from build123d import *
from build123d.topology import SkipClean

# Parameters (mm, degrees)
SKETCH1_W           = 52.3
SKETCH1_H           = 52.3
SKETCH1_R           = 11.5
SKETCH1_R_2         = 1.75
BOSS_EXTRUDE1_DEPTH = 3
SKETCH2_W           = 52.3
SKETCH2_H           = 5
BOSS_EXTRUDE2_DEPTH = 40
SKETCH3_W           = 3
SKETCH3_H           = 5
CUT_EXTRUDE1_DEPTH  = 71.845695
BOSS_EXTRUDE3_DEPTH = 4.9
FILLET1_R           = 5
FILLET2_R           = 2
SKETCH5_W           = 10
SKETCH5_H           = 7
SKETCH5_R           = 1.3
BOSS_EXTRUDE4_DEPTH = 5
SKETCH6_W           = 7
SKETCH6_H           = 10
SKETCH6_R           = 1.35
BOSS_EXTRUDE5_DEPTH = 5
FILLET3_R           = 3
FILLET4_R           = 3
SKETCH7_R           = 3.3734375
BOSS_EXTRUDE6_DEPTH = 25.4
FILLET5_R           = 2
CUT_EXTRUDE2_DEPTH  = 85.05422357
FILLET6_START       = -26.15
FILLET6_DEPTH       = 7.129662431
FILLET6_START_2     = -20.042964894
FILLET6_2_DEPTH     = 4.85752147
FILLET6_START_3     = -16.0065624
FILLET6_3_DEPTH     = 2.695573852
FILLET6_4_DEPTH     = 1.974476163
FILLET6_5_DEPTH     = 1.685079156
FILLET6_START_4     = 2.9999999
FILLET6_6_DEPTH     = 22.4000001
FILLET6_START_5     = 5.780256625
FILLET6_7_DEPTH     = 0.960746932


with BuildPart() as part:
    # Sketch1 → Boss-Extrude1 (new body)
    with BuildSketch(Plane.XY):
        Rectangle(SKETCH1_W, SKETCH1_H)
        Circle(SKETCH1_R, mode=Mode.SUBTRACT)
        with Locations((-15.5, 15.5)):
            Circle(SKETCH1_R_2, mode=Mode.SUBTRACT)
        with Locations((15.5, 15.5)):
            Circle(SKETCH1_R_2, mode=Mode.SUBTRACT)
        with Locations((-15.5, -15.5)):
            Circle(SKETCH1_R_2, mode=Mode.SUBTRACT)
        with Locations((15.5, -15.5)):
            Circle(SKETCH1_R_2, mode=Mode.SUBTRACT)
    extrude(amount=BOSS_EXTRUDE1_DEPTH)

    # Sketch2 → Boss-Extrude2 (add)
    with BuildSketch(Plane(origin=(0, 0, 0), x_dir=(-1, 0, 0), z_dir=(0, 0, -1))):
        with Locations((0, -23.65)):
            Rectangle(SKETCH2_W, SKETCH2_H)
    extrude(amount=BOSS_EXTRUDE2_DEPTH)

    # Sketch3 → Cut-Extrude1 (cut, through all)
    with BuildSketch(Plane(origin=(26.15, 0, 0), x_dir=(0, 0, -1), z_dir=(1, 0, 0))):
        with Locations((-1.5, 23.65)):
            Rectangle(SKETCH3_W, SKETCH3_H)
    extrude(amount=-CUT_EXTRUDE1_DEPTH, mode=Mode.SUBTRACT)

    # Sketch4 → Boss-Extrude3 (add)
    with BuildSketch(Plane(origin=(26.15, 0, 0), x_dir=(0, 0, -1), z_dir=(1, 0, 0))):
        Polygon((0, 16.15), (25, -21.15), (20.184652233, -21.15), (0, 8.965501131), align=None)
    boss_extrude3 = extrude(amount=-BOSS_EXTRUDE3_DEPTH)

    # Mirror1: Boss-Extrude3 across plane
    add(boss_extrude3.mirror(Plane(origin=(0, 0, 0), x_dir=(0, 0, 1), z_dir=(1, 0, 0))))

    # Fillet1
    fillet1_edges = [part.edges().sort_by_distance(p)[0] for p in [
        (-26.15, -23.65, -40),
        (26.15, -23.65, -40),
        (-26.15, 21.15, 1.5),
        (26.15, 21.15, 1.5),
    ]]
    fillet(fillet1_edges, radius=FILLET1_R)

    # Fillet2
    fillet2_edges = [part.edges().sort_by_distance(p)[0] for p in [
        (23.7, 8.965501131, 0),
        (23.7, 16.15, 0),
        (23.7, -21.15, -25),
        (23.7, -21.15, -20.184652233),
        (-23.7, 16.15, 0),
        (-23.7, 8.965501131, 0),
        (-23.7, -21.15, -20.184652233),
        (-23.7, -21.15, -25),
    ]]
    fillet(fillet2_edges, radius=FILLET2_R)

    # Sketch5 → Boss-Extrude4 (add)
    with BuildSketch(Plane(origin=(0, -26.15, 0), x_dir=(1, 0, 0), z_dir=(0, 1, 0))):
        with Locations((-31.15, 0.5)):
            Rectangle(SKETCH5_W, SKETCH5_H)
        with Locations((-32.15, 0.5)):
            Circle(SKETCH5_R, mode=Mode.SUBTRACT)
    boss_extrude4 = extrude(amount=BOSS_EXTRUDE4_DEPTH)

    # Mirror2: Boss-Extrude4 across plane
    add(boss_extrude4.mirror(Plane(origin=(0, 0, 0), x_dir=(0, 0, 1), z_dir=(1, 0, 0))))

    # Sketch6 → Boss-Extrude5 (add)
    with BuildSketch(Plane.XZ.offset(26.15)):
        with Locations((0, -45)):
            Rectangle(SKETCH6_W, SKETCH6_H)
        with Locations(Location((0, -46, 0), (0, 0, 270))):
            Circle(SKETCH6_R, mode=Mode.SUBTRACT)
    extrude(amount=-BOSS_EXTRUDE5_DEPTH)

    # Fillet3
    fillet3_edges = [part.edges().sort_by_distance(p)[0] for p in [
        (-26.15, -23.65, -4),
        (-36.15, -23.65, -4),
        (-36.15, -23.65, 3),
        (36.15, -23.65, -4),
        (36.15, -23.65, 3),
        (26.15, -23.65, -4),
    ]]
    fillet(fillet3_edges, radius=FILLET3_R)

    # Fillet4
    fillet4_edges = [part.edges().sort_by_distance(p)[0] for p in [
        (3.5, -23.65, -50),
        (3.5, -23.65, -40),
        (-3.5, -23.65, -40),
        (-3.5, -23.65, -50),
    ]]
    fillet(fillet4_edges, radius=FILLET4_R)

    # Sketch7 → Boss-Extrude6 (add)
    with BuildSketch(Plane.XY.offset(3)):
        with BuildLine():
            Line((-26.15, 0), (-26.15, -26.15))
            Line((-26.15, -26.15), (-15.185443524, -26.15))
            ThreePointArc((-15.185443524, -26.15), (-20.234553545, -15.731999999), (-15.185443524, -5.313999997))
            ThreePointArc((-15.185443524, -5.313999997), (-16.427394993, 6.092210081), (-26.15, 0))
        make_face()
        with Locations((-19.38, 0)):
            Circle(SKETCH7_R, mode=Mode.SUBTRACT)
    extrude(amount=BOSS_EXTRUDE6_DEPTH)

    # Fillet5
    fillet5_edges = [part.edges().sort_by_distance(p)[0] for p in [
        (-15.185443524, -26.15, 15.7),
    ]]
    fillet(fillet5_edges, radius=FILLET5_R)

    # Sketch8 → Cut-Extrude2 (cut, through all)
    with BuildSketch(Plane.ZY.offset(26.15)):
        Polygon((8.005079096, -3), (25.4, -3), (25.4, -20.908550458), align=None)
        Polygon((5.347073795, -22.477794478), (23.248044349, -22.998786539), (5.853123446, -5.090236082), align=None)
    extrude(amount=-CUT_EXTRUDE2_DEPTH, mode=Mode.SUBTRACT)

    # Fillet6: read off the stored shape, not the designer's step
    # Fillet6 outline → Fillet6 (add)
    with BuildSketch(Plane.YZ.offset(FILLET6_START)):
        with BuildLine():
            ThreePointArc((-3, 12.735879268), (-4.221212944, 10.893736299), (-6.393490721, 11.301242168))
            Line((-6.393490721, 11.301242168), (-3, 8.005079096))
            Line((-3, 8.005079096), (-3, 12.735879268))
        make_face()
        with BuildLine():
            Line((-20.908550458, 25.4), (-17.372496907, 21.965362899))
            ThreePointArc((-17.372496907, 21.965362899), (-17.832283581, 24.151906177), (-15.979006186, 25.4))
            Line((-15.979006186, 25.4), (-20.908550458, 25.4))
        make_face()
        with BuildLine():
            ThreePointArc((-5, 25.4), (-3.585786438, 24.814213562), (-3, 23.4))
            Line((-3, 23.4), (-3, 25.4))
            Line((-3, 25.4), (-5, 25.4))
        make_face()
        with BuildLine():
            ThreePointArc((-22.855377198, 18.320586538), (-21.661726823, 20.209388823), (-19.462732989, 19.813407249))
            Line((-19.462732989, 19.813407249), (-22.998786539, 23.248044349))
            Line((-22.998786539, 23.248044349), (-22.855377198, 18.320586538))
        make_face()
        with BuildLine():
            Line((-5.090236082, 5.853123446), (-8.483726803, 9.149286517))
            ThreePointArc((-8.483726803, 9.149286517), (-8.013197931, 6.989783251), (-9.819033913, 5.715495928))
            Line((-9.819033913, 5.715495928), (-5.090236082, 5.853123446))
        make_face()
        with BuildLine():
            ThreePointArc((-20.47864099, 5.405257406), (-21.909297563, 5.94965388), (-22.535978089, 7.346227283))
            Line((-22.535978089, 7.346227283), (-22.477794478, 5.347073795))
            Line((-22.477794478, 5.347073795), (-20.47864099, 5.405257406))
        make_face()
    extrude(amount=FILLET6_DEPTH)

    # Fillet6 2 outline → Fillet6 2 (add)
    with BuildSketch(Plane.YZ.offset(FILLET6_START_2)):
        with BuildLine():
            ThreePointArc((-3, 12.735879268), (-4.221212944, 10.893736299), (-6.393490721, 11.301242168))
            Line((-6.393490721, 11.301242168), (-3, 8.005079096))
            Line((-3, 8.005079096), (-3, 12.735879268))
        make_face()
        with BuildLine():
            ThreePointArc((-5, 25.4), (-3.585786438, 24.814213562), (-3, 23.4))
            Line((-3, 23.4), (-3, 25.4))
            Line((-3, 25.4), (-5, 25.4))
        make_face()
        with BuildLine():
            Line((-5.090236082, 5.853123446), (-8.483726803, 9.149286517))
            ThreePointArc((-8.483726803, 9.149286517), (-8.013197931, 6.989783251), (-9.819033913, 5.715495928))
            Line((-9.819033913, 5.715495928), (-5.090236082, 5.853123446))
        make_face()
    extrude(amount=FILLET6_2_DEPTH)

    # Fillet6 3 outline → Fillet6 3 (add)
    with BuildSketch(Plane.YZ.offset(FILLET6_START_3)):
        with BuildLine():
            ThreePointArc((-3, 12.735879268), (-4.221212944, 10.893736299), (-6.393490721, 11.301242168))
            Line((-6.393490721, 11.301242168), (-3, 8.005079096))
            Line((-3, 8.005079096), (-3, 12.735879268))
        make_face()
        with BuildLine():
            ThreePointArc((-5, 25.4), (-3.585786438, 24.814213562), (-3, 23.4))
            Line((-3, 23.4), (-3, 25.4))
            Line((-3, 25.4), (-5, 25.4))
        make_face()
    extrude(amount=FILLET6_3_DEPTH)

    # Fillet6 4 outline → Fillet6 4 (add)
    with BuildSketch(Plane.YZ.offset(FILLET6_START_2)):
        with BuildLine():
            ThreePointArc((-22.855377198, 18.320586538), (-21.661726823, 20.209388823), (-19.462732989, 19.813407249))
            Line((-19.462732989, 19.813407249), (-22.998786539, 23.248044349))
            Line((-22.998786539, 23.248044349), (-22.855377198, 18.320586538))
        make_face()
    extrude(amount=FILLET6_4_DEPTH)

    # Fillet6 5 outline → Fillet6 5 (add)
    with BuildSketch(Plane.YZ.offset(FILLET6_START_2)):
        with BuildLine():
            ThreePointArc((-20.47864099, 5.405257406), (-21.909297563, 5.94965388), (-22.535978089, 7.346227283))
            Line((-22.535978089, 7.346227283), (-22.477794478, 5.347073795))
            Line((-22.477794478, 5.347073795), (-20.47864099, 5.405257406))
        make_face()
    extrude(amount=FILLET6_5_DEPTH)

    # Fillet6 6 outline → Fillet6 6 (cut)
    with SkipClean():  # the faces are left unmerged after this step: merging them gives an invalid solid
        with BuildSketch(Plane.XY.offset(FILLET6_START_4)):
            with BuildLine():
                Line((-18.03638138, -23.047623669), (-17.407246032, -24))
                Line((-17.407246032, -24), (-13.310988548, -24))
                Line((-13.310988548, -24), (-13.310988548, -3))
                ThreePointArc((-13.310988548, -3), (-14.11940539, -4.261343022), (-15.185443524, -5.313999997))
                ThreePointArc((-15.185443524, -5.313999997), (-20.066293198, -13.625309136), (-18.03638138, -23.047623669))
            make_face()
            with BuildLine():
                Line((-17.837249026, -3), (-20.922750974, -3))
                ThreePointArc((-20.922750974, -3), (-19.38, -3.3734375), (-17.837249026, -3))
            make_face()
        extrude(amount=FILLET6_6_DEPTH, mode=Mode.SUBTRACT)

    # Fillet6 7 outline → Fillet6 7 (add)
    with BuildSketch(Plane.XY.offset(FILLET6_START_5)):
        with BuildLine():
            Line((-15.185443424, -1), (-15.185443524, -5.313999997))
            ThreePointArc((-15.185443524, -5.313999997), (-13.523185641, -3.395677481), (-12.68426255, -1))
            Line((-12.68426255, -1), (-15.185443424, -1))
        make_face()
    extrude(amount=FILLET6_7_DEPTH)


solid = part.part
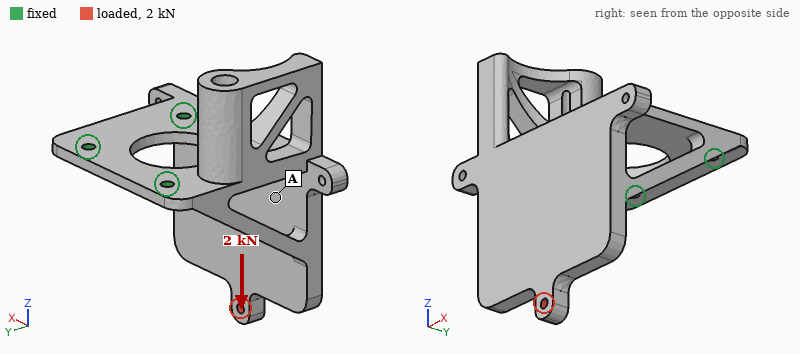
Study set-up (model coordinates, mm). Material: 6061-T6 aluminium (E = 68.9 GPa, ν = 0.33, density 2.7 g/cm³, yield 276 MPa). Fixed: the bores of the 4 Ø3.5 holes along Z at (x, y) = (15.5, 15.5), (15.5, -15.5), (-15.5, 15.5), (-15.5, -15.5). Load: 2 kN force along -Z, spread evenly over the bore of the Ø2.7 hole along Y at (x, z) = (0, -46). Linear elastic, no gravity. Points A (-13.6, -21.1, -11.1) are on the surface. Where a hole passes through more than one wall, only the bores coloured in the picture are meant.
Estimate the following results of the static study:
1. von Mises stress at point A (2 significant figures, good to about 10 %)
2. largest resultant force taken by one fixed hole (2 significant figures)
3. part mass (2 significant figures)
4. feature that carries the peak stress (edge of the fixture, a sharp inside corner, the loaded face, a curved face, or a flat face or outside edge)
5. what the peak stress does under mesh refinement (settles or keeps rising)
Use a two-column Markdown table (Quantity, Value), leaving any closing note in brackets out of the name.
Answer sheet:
| Quantity | Value |
|---|---|
| von Mises stress at point A | 20 MPa |
| largest resultant force taken by one fixed hole | 1.2 kN |
| part mass | 63 g |
| feature that carries the peak stress | edge of the fixture |
| what the peak stress does under mesh refinement | keeps rising |
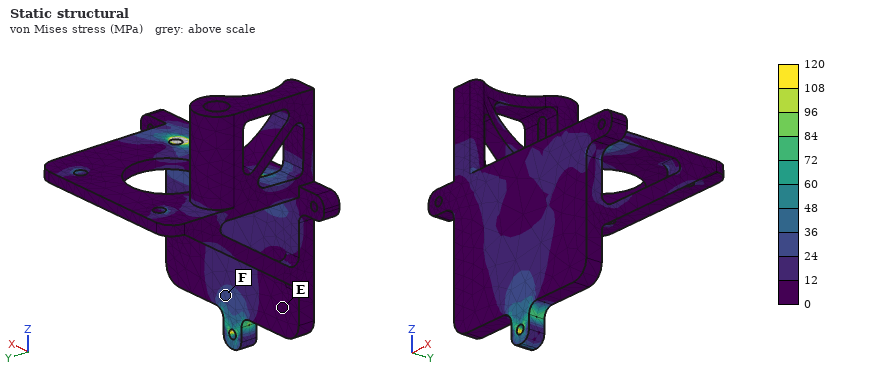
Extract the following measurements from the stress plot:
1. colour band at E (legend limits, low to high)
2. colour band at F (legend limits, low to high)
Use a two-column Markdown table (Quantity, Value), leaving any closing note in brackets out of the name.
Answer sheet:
| Quantity | Value |
|---|---|
| colour band at E | 0 to 12 MPa |
| colour band at F | 24 to 36 MPa |
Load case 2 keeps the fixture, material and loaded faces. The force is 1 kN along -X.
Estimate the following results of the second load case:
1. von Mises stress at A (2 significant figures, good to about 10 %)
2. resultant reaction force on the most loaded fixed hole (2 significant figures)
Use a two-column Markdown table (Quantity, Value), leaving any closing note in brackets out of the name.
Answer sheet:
| Quantity | Value |
|---|---|
| von Mises stress at A | 27 MPa |
| resultant reaction force on the most loaded fixed hole | 1.6 kN |
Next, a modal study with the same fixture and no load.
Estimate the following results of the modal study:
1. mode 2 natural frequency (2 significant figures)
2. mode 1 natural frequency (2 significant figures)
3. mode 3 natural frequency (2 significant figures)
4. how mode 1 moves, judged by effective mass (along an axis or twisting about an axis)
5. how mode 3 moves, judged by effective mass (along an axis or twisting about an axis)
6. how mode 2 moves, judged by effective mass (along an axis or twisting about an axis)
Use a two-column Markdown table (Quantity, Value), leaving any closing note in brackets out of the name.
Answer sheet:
| Quantity | Value |
|---|---|
| mode 2 natural frequency | 3600 Hz |
| mode 1 natural frequency | 3100 Hz |
| mode 3 natural frequency | 4500 Hz |
| how mode 1 moves, judged by effective mass | along Y |
| how mode 3 moves, judged by effective mass | along X |
| how mode 2 moves, judged by effective mass | twisting about Y |
